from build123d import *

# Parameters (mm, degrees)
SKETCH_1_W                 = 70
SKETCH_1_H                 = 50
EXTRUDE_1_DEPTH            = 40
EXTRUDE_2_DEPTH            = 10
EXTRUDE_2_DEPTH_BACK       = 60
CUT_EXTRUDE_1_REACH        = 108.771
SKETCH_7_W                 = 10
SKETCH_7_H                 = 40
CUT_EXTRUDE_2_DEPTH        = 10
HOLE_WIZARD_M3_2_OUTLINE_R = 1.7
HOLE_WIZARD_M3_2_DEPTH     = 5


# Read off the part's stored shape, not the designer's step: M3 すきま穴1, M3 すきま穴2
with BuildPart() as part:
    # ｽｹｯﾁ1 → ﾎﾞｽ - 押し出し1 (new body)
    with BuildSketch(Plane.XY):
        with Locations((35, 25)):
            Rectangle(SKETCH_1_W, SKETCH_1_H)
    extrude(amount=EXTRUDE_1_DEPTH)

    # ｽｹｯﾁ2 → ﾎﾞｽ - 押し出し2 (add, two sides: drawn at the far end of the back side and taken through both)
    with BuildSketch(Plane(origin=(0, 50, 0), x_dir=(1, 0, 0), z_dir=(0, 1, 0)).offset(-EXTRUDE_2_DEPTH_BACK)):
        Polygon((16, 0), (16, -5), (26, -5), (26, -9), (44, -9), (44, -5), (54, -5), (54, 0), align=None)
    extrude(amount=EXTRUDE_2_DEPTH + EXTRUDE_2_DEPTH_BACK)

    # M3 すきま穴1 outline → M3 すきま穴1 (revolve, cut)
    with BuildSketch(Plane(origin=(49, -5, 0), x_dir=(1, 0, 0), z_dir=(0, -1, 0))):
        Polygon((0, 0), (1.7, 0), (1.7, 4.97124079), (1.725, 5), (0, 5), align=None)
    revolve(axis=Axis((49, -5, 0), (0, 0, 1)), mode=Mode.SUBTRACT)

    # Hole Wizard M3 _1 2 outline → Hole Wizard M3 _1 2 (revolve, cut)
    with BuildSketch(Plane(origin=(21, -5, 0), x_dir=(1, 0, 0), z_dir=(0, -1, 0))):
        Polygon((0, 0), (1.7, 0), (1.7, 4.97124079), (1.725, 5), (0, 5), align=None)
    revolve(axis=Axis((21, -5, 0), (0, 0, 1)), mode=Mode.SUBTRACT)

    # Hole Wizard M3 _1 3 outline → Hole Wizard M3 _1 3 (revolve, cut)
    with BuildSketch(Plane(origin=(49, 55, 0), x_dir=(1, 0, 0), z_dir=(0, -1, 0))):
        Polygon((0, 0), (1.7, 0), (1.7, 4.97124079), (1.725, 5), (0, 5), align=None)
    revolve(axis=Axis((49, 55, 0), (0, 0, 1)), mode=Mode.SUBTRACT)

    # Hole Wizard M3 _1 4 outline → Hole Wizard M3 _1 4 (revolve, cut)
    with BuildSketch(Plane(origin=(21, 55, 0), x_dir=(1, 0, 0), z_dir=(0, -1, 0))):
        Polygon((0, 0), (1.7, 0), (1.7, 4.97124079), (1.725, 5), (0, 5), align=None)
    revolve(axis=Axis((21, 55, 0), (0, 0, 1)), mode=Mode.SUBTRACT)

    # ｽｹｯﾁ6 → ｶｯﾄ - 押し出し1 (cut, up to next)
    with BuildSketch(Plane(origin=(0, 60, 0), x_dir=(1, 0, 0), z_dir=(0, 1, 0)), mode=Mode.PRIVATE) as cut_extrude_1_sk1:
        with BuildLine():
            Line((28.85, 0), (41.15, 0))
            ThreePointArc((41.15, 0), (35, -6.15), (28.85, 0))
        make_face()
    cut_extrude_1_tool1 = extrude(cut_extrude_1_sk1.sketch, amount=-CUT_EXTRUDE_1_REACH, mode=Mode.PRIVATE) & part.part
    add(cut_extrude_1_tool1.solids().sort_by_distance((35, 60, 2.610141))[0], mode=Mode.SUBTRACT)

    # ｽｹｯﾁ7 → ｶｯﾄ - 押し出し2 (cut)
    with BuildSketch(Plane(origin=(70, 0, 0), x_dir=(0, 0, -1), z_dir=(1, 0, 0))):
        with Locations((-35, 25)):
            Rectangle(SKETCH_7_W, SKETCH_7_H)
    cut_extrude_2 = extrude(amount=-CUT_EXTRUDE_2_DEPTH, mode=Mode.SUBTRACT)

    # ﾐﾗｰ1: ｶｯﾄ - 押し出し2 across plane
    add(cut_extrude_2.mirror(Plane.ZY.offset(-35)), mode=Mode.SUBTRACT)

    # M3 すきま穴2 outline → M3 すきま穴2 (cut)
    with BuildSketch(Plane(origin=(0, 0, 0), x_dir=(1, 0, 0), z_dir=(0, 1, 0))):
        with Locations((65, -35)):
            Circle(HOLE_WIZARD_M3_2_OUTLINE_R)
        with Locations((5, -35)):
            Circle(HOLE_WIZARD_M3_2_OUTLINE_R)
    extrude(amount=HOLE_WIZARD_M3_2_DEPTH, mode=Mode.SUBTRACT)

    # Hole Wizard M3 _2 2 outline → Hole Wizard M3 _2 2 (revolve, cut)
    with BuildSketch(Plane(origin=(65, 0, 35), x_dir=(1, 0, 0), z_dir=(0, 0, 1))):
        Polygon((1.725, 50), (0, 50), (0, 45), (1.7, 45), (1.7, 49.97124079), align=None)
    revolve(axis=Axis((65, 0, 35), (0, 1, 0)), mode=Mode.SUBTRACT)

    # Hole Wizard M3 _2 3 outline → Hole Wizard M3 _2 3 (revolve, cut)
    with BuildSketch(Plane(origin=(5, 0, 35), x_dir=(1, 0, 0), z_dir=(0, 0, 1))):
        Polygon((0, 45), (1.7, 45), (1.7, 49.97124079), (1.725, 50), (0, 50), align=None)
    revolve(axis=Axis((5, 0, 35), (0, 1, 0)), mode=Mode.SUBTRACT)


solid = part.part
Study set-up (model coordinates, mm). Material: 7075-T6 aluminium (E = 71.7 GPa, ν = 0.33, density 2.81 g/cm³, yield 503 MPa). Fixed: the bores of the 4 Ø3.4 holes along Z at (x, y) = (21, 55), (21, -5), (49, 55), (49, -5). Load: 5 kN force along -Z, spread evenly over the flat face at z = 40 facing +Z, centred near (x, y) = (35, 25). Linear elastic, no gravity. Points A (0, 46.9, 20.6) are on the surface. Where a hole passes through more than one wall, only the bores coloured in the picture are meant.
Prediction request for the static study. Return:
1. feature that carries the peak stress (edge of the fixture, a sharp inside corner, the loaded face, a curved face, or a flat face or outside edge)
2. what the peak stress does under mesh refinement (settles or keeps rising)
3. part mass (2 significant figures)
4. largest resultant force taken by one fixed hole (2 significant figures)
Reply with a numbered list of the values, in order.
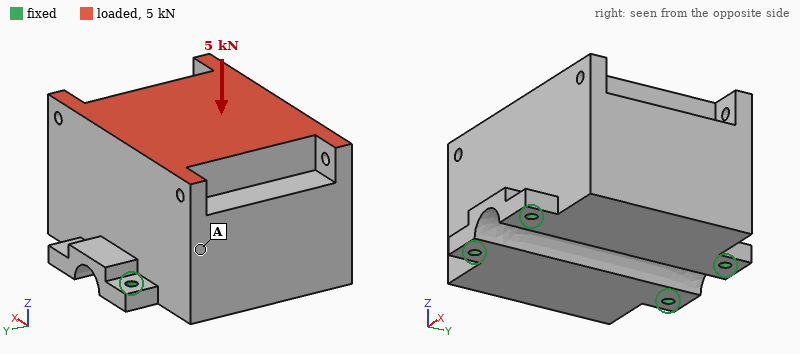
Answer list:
1. edge of the fixture
2. keeps rising
3. 370 g
4. 1.4 kN
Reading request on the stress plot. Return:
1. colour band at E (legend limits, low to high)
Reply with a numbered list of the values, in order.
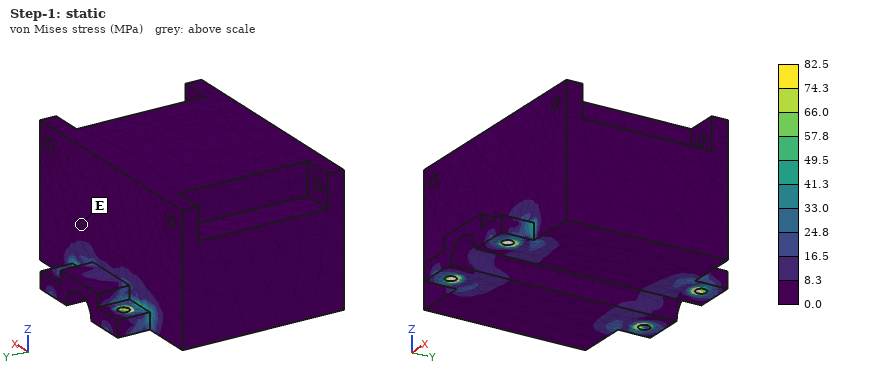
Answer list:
1. 0.0 to 8.3 MPa
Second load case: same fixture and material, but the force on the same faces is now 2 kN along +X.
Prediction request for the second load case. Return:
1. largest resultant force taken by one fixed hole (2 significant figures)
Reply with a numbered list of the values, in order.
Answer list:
1. 1.5 kN
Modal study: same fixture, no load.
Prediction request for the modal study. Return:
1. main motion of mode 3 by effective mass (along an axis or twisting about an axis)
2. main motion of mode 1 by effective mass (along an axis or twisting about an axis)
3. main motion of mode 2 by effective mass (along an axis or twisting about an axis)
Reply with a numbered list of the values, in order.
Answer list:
1. along Y
2. along X
3. along Z
